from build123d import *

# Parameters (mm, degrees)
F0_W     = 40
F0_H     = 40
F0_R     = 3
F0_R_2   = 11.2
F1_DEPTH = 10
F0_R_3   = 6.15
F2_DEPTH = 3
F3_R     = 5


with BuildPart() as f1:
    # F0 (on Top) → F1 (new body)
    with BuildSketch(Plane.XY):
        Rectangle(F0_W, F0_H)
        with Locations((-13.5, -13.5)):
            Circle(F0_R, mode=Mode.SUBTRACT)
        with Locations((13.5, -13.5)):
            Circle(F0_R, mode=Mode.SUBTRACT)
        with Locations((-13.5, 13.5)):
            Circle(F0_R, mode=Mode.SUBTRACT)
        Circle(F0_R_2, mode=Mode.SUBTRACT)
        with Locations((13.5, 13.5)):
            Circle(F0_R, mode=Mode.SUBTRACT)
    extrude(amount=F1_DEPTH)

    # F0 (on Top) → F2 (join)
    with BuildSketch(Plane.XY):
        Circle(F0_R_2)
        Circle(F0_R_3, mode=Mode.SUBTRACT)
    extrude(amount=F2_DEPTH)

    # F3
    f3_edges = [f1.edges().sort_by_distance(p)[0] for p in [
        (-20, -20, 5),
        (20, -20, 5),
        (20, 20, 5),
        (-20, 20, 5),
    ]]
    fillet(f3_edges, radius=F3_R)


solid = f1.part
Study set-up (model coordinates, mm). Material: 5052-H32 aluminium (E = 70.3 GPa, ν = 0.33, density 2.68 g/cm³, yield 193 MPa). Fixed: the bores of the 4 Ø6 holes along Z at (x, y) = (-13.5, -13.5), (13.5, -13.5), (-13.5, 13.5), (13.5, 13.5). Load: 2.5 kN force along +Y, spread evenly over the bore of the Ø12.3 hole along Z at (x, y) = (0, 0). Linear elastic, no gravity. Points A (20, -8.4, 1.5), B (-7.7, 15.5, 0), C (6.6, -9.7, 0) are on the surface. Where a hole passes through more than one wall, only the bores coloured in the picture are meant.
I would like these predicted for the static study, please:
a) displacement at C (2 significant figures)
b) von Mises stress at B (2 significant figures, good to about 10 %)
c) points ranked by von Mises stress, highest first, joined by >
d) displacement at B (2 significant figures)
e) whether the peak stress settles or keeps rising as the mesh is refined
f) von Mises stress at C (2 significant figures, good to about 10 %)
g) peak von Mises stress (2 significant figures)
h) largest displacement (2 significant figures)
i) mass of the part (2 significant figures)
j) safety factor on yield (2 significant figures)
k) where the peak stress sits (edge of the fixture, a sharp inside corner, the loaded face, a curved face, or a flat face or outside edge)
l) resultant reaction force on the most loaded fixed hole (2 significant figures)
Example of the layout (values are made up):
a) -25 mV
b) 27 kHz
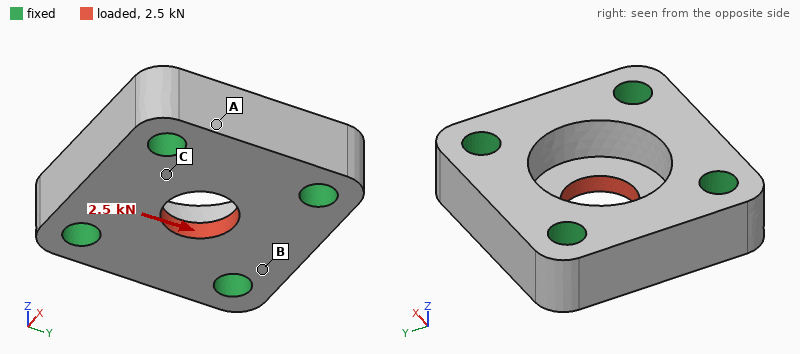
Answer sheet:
a) 1.8 µm
b) 12 MPa
c) C > B > A
d) 1.1 µm
e) settles
f) 18 MPa
g) 38 MPa
h) 4.4 µm
i) 31 g
j) 5.0
k) the loaded face
l) 660 N
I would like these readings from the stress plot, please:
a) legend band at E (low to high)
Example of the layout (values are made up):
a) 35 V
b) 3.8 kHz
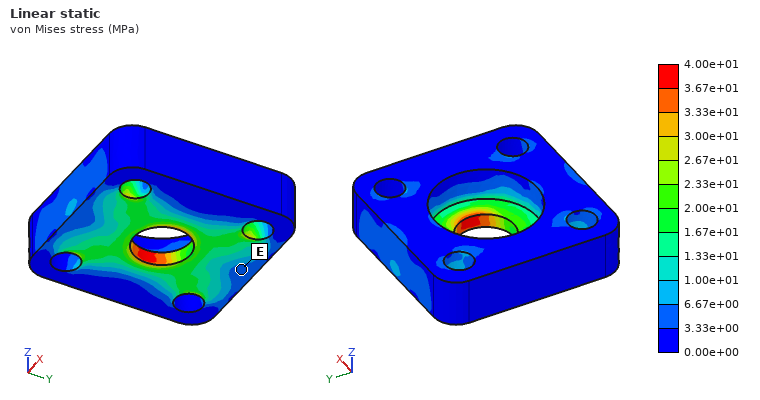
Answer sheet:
a) 3.33e+00 to 6.67e+00 MPa
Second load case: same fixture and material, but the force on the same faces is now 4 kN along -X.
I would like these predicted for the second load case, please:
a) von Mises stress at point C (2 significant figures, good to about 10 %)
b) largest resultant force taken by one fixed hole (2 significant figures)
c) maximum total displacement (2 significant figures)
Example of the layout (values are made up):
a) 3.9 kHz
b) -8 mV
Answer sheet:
a) 22 MPa
b) 1.1 kN
c) 7.1 µm
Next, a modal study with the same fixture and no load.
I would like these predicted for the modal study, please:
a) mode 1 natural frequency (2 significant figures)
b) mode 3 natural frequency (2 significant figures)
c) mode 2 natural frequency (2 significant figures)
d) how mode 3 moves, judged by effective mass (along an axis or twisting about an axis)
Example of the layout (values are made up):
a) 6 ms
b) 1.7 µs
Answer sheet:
a) 49 kHz
b) 53 kHz
c) 49 kHz
d) twisting about X
